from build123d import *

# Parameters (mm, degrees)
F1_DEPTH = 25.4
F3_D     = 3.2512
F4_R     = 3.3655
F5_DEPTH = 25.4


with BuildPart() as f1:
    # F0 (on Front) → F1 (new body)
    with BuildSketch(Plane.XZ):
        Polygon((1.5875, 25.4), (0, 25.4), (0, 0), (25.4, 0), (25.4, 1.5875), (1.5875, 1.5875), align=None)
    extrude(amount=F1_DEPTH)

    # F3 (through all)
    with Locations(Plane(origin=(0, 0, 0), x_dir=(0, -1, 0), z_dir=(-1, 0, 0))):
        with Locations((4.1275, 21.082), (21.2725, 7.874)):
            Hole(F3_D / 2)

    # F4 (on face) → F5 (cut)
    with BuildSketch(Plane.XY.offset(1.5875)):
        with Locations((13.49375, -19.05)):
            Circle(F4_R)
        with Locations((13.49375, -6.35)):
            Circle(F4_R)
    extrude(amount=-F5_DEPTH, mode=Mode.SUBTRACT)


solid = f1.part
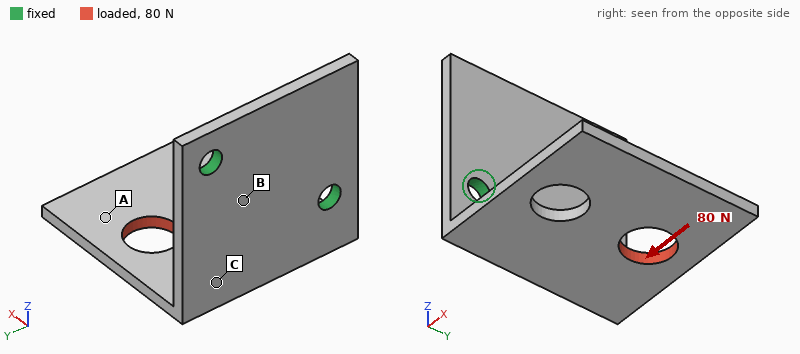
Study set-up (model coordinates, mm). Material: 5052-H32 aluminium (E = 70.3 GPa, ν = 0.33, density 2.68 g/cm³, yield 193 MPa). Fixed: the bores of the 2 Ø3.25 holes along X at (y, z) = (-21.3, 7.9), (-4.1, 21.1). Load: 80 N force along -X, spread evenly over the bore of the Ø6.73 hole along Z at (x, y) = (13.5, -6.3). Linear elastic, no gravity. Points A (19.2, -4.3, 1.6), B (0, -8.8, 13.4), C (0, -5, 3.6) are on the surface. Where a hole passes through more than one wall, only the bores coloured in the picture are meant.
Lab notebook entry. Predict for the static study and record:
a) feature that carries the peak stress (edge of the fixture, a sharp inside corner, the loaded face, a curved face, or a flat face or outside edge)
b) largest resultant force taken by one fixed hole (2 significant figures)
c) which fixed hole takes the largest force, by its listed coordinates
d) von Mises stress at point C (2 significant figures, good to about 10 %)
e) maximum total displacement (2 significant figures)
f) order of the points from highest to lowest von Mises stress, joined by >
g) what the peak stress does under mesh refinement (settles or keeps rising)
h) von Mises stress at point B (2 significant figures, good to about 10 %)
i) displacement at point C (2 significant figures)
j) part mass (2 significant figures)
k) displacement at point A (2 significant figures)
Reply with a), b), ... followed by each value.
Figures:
a) edge of the fixture
b) 61 N
c) (-21.3, 7.9)
d) 27 MPa
e) 0.33 mm
f) B > C > A
g) keeps rising
h) 44 MPa
i) 0.11 mm
j) 4.9 g
k) 0.25 mm
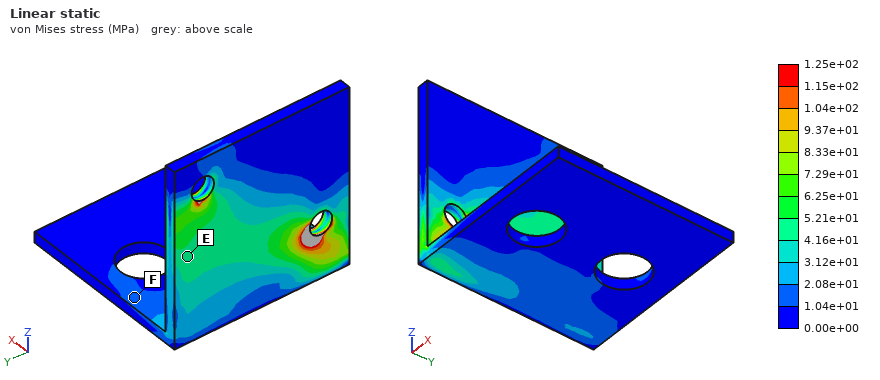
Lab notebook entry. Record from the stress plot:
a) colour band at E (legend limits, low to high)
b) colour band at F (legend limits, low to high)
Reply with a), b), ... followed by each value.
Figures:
a) 4.16e+01 to 5.21e+01 MPa
b) 1.04e+01 to 2.08e+01 MPa
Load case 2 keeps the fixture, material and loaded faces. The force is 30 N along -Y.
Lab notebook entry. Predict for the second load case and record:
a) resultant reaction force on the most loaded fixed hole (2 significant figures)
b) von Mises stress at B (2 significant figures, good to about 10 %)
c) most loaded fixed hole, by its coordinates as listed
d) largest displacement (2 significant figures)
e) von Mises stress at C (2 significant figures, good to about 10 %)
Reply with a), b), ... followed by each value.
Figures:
a) 31 N
b) 13 MPa
c) (-21.3, 7.9)
d) 92 µm
e) 9.4 MPa
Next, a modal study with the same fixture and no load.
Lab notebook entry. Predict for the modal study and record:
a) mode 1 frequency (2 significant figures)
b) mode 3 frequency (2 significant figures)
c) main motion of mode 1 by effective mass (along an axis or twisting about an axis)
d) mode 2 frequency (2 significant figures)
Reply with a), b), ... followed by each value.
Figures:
a) 1400 Hz
b) 4500 Hz
c) along Z
d) 2400 Hz
